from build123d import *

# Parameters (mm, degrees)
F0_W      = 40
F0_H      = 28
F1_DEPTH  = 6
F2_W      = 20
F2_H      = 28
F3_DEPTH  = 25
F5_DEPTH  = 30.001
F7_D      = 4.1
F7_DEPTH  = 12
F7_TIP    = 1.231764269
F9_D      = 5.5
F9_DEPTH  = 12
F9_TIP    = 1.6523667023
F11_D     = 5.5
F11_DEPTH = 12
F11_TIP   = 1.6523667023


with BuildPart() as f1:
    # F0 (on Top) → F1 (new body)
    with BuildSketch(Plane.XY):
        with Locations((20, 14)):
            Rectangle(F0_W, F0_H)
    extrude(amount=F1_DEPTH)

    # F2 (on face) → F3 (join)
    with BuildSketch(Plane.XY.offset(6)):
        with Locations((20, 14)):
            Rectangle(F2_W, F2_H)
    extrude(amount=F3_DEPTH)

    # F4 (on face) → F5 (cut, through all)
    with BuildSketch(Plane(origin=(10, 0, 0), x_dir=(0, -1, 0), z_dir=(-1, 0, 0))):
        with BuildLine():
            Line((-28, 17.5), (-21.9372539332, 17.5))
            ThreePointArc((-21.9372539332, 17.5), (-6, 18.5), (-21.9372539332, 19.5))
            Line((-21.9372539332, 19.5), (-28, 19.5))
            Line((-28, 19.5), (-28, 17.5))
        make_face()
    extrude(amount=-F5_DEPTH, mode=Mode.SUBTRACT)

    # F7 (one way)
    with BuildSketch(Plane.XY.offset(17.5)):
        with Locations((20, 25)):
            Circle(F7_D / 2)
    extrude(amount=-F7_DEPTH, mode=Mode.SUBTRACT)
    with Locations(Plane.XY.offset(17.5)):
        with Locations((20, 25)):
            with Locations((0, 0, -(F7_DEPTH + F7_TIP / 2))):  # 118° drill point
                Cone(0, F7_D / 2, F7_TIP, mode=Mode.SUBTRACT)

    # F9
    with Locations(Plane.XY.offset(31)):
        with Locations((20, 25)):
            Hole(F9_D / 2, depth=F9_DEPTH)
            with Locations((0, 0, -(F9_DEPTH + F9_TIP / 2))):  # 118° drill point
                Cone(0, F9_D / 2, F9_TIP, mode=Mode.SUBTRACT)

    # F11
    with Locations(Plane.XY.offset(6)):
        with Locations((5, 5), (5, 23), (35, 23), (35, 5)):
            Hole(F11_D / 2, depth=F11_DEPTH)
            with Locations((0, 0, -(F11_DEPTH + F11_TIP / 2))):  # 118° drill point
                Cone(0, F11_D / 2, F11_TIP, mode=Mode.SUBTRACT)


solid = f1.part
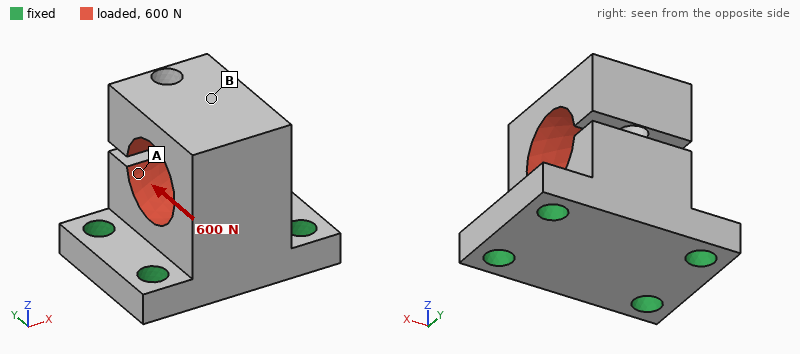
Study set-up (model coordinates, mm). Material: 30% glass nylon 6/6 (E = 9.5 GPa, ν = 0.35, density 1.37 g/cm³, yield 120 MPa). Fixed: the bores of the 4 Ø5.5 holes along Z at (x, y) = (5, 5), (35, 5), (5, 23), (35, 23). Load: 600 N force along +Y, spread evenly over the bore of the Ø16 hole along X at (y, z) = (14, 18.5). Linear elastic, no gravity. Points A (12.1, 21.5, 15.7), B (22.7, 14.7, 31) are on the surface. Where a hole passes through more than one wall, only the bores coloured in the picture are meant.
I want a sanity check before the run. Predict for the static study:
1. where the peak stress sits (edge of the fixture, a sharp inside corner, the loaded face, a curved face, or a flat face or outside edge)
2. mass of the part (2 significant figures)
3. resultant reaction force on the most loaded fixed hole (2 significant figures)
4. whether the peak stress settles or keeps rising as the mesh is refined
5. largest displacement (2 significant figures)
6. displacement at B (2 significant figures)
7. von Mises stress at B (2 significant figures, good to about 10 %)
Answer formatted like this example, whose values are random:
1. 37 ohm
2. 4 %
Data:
1. edge of the fixture
2. 21 g
3. 310 N
4. keeps rising
5. 0.20 mm
6. 0.17 mm
7. 6.6 MPa
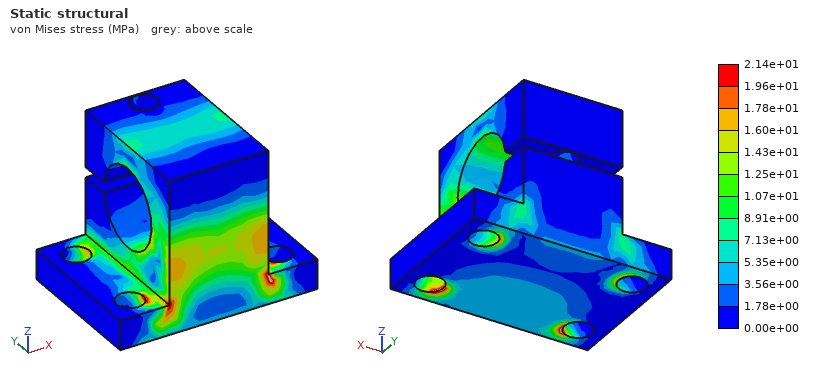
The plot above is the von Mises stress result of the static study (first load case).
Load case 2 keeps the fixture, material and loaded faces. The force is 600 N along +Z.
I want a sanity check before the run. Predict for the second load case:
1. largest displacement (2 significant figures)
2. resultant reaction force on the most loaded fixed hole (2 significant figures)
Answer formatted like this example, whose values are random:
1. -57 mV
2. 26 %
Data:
1. 0.39 mm
2. 170 N
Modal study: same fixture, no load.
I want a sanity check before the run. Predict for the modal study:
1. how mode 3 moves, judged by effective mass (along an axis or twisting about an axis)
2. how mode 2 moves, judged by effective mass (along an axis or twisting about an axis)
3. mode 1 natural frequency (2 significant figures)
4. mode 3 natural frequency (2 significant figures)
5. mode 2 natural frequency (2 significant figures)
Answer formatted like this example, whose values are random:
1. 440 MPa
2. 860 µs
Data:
1. along Y
2. along X
3. 1900 Hz
4. 4000 Hz
5. 2600 Hz
